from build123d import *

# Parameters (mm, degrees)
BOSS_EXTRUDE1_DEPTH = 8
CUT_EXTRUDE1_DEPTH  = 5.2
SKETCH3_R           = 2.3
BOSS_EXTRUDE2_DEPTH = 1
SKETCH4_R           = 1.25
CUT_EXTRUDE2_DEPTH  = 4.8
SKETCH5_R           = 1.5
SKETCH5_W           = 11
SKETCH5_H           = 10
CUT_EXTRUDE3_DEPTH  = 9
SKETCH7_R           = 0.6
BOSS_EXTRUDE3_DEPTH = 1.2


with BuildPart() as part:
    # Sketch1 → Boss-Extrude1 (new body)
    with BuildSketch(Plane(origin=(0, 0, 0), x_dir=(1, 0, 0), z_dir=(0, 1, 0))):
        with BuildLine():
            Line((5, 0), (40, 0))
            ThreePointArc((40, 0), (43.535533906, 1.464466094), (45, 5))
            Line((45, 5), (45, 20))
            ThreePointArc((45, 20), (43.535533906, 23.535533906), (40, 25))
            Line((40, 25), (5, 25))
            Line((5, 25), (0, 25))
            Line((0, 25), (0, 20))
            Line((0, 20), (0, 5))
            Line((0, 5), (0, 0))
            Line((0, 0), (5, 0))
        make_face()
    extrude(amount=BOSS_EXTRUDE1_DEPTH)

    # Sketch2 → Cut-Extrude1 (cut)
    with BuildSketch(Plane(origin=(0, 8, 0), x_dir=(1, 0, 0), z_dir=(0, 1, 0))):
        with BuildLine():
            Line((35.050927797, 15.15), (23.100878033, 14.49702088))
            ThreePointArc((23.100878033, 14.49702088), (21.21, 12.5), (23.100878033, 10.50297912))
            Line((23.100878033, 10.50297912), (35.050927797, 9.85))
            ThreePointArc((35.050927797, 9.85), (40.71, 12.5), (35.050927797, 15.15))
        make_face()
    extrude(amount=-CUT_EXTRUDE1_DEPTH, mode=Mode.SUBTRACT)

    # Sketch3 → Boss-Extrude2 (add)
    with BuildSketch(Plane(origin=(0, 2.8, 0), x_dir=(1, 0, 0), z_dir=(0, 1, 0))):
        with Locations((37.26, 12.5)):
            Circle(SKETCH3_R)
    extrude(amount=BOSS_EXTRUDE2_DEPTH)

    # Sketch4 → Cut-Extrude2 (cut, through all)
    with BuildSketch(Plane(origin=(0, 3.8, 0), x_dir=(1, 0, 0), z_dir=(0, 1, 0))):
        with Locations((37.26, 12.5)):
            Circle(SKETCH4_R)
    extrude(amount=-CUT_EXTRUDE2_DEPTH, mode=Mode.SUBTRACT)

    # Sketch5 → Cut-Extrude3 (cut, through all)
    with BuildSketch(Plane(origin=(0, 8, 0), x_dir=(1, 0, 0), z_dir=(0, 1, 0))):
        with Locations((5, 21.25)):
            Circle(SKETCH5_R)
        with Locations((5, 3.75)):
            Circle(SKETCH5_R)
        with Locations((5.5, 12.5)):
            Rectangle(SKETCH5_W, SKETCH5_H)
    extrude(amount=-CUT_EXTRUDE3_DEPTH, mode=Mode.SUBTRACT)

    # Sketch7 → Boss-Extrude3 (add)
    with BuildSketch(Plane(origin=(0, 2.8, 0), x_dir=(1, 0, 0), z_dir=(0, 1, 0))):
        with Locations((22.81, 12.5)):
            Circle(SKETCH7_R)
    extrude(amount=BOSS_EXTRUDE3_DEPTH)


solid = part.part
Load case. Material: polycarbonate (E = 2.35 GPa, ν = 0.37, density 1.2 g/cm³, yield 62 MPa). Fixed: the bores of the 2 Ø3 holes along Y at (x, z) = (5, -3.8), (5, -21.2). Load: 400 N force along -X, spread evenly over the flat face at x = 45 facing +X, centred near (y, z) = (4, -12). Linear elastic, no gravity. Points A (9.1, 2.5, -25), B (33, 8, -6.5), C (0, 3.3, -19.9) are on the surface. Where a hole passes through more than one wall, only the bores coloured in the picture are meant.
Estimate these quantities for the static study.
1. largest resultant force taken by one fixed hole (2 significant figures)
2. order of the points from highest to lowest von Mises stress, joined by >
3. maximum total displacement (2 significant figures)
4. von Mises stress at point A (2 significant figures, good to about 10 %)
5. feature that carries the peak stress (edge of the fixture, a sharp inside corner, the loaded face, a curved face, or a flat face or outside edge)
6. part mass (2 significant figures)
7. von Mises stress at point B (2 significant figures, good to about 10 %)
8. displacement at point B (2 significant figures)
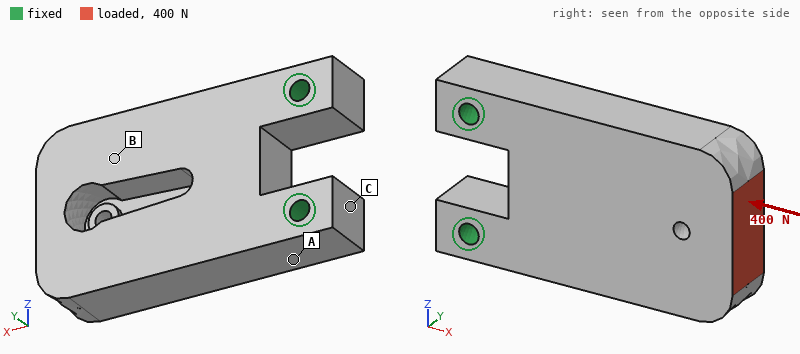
200 N
B > A > C
70 µm
2.1 MPa
a curved face
8.9 g
3.6 MPa
35 µm
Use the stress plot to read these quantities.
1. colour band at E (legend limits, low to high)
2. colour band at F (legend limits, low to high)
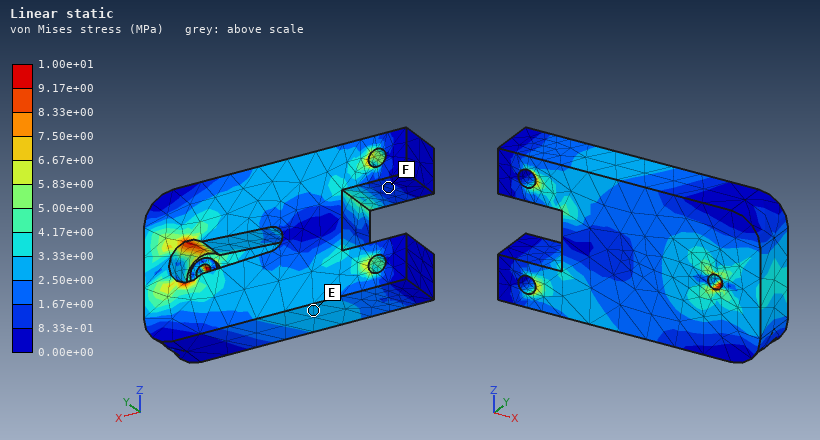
2.50e+00 to 3.33e+00 MPa
8.33e-01 to 1.67e+00 MPa
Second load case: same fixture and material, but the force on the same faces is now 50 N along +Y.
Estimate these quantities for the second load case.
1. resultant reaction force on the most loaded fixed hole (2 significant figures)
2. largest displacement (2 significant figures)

25 N
0.61 mm
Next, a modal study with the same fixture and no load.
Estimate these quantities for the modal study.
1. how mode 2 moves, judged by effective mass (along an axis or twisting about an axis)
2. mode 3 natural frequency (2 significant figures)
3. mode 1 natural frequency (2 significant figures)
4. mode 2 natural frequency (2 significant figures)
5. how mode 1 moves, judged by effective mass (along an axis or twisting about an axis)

along Z
3000 Hz
990 Hz
2600 Hz
along Y
